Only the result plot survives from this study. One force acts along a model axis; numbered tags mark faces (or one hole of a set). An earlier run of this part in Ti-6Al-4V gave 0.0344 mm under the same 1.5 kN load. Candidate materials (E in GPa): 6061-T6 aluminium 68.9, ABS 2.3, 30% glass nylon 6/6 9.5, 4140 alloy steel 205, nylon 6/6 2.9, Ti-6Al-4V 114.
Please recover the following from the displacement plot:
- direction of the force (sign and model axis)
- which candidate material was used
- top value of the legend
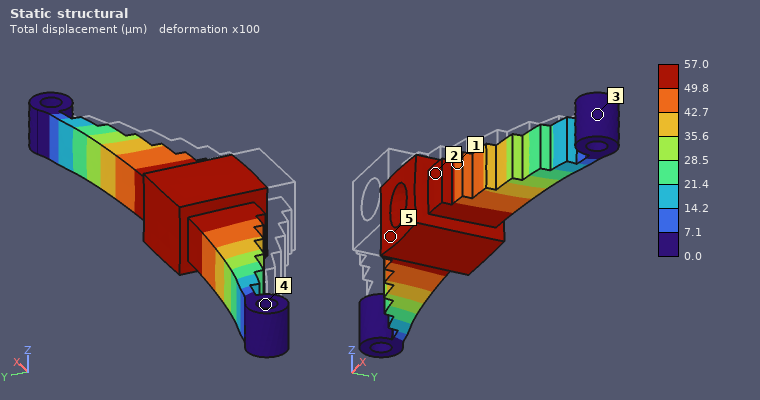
+Y
6061-T6 aluminium
57.0 µm
